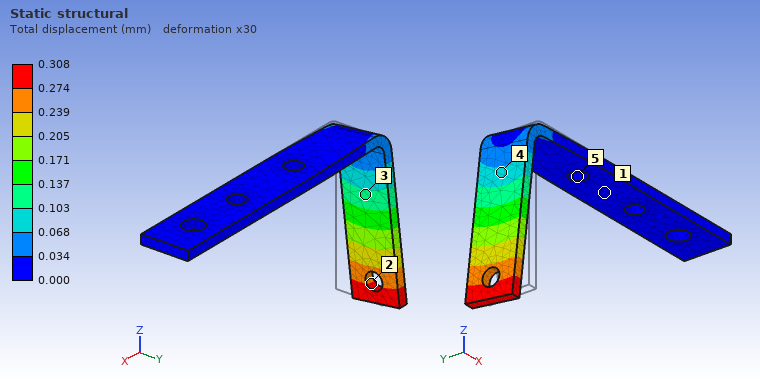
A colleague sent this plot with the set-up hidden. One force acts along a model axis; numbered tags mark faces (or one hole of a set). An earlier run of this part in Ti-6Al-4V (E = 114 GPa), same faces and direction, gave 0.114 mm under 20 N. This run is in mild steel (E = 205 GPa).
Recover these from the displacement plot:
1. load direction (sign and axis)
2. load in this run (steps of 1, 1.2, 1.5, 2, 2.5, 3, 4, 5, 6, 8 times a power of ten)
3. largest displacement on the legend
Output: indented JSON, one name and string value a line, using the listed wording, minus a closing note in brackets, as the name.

{
  "load direction": "+Y",
  "load in this run": "100 N",
  "largest displacement on the legend": "0.308 mm"
}
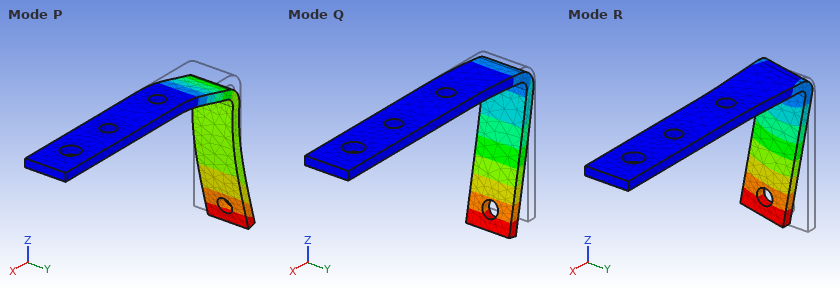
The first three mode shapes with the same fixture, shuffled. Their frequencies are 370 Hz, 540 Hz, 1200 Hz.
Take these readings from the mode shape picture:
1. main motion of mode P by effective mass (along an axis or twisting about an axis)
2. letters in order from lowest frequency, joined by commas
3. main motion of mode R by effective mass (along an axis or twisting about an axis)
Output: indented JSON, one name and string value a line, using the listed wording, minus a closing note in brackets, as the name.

{
  "main motion of mode P by effective mass": "along Z",
  "letters in order from lowest frequency, joined by commas": "Q, R, P",
  "main motion of mode R by effective mass": "along Y"
}
